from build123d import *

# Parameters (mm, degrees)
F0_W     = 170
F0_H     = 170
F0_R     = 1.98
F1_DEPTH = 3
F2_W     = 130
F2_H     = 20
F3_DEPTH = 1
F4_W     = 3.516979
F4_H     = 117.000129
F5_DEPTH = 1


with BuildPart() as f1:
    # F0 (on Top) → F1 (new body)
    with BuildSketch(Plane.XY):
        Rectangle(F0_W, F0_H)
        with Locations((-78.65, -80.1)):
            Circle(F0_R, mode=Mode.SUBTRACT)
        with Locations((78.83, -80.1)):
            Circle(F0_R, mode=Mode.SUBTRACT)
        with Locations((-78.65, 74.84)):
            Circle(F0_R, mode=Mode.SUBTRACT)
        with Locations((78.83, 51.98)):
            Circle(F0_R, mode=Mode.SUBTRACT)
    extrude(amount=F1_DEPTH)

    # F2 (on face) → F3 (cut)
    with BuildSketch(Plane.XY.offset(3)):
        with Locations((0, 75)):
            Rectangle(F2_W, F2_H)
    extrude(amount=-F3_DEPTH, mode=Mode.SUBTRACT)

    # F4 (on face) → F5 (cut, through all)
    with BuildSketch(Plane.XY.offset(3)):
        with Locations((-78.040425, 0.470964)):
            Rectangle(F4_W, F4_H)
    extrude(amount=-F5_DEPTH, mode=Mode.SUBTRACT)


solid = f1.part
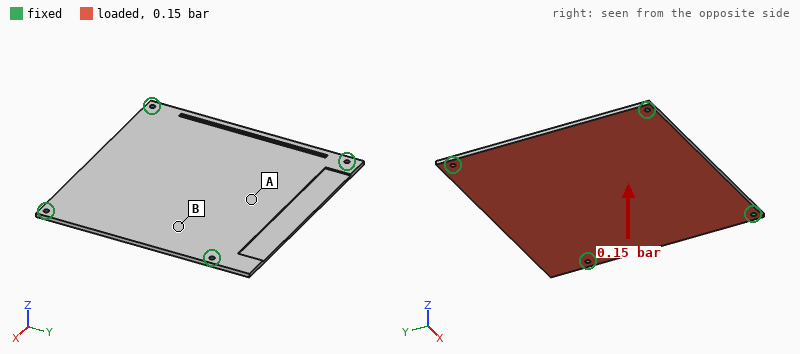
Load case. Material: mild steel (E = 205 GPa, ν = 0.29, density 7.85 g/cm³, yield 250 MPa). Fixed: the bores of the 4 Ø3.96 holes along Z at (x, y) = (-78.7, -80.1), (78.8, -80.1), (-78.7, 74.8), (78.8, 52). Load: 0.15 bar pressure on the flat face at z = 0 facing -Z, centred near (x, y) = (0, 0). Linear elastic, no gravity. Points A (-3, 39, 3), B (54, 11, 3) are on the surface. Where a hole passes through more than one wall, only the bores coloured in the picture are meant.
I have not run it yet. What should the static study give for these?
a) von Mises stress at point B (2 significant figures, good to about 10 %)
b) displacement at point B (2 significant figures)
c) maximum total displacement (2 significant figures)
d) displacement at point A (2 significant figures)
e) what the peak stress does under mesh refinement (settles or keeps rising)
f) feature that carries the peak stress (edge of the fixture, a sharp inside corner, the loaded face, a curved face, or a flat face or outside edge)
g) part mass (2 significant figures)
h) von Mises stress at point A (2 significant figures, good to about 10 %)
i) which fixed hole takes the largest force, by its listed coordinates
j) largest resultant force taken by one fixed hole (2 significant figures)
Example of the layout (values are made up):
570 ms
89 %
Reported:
8.0 MPa
0.077 mm
0.15 mm
0.13 mm
keeps rising
edge of the fixture
660 g
16 MPa
(78.8, 52)
140 N
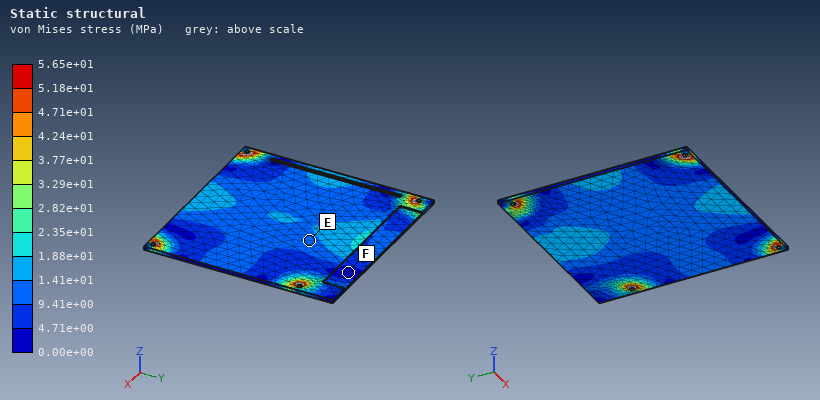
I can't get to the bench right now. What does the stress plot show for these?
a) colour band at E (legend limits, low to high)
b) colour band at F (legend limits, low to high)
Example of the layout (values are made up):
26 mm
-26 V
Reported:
9.41e+00 to 1.41e+01 MPa
0.00e+00 to 4.71e+00 MPa
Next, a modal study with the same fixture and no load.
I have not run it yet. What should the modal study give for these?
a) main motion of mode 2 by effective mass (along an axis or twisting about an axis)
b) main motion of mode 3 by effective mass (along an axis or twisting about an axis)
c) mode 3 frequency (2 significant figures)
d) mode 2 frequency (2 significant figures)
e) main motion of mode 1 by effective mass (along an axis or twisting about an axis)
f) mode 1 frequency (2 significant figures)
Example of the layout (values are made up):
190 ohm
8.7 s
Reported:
twisting about X
twisting about Y
730 Hz
650 Hz
along Z
390 Hz
